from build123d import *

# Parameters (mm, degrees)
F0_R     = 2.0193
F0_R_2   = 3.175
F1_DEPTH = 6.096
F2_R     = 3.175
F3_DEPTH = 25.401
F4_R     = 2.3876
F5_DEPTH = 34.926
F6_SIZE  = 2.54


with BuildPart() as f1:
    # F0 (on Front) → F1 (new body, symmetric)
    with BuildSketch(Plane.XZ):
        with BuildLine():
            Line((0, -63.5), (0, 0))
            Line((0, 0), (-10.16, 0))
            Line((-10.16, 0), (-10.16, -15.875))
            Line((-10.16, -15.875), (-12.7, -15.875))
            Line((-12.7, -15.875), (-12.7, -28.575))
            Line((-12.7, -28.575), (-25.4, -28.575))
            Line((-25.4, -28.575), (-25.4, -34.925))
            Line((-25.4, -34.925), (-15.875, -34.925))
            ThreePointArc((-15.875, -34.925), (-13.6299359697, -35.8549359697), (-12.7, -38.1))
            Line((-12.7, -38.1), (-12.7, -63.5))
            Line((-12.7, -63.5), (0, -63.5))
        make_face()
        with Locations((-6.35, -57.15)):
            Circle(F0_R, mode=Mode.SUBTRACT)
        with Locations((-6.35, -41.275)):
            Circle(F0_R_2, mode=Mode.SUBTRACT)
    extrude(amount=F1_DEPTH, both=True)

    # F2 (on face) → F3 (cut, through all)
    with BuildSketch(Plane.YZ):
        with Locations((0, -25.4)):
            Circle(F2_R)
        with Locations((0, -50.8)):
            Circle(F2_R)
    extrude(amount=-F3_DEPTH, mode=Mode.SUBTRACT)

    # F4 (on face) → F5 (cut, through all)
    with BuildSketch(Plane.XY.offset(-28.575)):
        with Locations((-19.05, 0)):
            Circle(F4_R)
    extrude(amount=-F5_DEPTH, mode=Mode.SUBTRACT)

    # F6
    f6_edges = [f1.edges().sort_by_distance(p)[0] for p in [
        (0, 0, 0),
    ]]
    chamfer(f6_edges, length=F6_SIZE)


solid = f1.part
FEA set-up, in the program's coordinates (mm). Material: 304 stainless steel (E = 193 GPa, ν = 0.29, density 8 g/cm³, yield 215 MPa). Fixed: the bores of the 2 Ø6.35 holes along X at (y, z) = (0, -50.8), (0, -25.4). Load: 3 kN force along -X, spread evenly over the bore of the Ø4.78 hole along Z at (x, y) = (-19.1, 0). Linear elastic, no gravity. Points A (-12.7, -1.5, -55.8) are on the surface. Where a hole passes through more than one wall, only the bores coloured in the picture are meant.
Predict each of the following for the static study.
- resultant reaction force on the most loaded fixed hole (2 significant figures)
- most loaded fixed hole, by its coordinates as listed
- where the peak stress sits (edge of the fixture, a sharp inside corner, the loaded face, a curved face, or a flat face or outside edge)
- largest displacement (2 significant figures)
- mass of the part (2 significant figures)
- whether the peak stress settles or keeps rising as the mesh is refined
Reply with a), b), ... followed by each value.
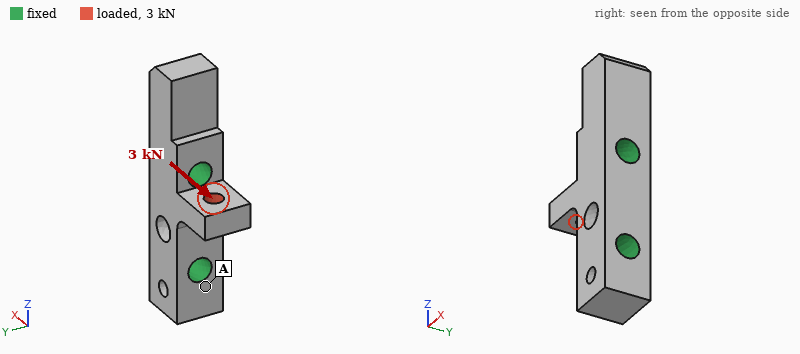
a) 2.6 kN
b) (0, -25.4)
c) edge of the fixture
d) 4.6 µm
e) 71 g
f) keeps rising
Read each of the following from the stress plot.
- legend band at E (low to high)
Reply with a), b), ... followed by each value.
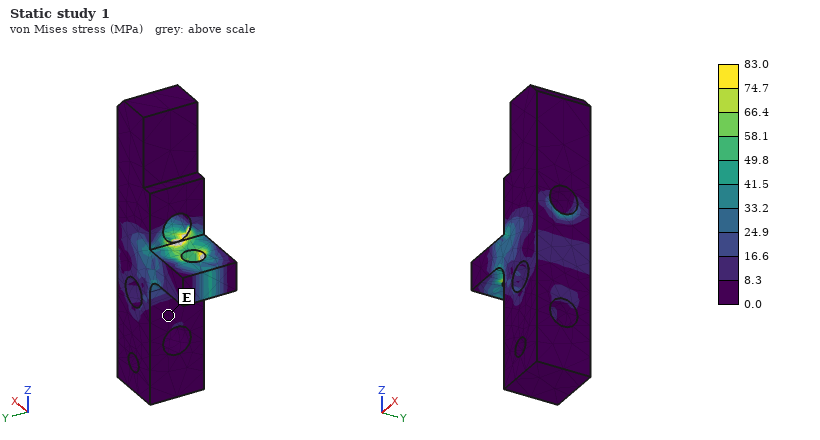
a) 0.0 to 8.3 MPa
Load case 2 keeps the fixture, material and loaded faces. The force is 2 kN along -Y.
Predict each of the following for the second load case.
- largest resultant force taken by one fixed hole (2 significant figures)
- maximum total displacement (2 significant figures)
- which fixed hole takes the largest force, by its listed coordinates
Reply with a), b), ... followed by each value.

a) 1.8 kN
b) 17 µm
c) (0, -25.4)
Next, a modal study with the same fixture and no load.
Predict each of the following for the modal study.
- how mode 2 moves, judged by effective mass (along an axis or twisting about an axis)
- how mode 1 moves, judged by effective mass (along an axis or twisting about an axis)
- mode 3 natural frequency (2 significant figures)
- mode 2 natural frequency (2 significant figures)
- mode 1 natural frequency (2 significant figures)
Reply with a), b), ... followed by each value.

a) along X
b) along Y
c) 22 kHz
d) 16 kHz
e) 14 kHz
